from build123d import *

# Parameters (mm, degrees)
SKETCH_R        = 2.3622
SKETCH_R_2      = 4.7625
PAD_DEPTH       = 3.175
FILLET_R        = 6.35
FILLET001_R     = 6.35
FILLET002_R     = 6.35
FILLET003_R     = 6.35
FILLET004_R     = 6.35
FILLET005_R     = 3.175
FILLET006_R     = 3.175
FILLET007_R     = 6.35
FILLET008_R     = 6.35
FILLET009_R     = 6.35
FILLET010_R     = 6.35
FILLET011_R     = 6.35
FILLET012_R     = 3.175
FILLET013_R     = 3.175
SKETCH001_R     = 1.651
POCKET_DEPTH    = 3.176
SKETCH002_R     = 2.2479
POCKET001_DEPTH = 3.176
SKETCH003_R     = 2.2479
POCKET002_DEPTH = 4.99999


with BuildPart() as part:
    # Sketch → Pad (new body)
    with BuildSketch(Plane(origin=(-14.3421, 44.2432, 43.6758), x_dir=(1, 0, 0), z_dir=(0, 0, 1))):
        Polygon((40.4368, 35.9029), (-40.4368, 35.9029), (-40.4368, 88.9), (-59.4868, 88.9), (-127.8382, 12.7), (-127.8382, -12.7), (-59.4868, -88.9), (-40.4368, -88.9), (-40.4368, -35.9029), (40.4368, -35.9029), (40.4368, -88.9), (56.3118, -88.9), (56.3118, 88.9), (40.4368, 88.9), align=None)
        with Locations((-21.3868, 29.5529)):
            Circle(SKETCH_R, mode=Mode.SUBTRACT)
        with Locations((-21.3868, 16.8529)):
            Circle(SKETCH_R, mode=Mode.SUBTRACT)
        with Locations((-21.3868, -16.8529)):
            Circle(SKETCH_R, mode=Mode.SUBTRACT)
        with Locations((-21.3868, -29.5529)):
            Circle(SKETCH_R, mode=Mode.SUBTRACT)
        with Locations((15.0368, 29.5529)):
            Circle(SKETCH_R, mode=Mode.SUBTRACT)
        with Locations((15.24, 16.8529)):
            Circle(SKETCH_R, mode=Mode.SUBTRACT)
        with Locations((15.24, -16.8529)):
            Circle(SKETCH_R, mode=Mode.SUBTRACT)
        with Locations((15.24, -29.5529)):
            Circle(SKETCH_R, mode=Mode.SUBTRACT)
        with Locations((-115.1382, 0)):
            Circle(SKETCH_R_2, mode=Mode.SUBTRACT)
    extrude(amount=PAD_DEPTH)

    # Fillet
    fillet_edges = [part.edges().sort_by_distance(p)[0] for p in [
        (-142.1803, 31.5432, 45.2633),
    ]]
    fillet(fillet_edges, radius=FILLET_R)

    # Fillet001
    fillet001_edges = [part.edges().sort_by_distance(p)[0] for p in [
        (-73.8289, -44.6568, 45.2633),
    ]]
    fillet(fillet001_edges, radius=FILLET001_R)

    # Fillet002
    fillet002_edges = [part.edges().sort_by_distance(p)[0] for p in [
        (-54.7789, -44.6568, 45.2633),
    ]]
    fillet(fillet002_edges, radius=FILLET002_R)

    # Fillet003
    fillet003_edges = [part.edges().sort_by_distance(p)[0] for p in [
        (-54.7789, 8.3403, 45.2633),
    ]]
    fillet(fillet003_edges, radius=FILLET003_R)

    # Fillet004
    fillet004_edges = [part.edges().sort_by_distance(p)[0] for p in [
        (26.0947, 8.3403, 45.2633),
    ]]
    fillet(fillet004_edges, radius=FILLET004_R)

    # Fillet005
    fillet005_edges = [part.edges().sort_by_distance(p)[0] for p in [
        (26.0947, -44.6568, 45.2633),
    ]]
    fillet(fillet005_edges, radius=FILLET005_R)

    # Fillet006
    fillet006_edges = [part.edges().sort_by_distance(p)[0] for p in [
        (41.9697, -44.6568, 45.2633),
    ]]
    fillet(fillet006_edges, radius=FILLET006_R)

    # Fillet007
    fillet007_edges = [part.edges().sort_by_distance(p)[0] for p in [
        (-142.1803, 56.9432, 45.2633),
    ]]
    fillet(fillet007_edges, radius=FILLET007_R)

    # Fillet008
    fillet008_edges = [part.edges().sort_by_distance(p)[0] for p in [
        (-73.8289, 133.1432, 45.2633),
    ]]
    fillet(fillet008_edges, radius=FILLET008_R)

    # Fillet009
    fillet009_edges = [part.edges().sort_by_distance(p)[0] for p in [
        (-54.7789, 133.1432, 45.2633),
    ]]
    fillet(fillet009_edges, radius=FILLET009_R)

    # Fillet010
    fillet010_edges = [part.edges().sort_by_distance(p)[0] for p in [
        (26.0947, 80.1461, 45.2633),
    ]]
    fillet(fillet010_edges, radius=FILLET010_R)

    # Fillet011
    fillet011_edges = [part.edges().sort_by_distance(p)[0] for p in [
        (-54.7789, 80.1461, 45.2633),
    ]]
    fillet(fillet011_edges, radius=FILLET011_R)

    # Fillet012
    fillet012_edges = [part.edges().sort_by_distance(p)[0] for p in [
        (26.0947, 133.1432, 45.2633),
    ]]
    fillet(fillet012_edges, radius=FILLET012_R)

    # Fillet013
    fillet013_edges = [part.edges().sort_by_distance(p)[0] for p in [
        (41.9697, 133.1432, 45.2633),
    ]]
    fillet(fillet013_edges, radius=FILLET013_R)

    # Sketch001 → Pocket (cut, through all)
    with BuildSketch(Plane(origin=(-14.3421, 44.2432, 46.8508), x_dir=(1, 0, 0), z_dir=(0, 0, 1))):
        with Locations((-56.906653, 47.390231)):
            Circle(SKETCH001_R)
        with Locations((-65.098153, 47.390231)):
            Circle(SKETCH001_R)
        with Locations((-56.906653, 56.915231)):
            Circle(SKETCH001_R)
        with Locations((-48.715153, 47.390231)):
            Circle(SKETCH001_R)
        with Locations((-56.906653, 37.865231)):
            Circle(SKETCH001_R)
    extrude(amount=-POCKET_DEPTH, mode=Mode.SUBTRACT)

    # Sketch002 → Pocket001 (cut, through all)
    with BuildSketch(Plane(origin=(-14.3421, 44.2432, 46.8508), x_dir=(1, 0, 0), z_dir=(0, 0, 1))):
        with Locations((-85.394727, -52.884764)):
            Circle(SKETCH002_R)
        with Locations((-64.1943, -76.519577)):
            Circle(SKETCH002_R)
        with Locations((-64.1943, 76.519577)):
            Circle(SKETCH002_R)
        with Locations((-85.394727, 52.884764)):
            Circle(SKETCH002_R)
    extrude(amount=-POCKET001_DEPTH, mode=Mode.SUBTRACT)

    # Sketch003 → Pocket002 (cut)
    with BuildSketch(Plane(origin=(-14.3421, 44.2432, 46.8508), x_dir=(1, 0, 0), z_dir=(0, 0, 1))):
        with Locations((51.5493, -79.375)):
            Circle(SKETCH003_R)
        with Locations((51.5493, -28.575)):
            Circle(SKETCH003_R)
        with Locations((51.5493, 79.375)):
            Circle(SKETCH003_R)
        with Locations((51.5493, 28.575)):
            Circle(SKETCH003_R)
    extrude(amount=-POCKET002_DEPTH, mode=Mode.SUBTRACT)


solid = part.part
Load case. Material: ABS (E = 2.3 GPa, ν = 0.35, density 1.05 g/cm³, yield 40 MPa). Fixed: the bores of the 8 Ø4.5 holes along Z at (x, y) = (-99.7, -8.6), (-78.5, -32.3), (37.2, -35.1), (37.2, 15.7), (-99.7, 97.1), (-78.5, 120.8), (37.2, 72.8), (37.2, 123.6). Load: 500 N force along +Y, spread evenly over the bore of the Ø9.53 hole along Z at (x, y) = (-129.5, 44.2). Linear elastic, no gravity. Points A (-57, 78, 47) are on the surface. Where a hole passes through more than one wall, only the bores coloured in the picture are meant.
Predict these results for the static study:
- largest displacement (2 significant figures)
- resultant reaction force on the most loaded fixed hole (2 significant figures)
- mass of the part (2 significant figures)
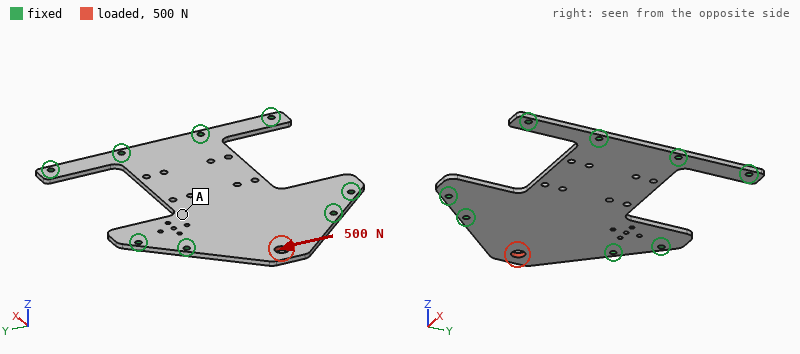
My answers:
0.15 mm
240 N
62 g
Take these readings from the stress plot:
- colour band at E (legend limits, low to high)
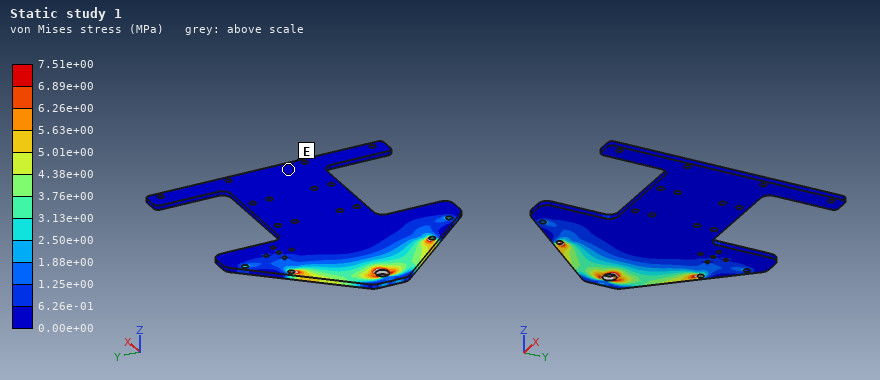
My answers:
0.00e+00 to 6.26e-01 MPa
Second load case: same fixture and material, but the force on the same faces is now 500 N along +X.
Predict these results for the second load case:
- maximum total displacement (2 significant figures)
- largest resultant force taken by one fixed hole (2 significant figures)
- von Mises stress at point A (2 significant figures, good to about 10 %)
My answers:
0.14 mm
170 N
0.84 MPa
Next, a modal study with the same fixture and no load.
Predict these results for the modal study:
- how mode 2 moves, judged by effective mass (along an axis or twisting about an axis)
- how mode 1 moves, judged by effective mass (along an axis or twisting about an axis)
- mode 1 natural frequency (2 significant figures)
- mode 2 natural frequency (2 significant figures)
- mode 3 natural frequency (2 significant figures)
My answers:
along Z
along Z
240 Hz
290 Hz
490 Hz
